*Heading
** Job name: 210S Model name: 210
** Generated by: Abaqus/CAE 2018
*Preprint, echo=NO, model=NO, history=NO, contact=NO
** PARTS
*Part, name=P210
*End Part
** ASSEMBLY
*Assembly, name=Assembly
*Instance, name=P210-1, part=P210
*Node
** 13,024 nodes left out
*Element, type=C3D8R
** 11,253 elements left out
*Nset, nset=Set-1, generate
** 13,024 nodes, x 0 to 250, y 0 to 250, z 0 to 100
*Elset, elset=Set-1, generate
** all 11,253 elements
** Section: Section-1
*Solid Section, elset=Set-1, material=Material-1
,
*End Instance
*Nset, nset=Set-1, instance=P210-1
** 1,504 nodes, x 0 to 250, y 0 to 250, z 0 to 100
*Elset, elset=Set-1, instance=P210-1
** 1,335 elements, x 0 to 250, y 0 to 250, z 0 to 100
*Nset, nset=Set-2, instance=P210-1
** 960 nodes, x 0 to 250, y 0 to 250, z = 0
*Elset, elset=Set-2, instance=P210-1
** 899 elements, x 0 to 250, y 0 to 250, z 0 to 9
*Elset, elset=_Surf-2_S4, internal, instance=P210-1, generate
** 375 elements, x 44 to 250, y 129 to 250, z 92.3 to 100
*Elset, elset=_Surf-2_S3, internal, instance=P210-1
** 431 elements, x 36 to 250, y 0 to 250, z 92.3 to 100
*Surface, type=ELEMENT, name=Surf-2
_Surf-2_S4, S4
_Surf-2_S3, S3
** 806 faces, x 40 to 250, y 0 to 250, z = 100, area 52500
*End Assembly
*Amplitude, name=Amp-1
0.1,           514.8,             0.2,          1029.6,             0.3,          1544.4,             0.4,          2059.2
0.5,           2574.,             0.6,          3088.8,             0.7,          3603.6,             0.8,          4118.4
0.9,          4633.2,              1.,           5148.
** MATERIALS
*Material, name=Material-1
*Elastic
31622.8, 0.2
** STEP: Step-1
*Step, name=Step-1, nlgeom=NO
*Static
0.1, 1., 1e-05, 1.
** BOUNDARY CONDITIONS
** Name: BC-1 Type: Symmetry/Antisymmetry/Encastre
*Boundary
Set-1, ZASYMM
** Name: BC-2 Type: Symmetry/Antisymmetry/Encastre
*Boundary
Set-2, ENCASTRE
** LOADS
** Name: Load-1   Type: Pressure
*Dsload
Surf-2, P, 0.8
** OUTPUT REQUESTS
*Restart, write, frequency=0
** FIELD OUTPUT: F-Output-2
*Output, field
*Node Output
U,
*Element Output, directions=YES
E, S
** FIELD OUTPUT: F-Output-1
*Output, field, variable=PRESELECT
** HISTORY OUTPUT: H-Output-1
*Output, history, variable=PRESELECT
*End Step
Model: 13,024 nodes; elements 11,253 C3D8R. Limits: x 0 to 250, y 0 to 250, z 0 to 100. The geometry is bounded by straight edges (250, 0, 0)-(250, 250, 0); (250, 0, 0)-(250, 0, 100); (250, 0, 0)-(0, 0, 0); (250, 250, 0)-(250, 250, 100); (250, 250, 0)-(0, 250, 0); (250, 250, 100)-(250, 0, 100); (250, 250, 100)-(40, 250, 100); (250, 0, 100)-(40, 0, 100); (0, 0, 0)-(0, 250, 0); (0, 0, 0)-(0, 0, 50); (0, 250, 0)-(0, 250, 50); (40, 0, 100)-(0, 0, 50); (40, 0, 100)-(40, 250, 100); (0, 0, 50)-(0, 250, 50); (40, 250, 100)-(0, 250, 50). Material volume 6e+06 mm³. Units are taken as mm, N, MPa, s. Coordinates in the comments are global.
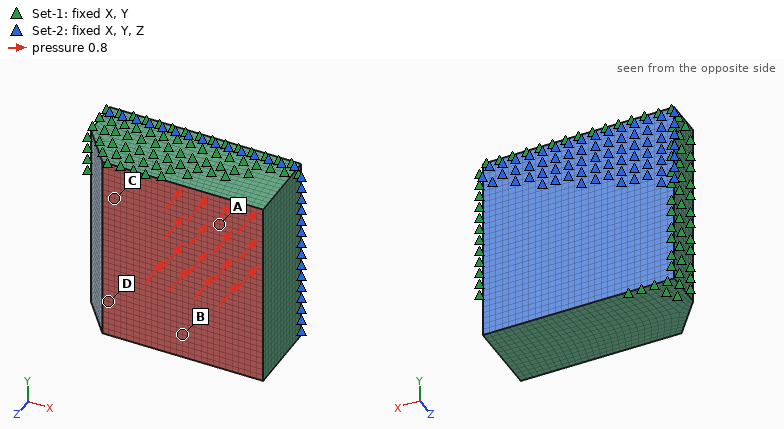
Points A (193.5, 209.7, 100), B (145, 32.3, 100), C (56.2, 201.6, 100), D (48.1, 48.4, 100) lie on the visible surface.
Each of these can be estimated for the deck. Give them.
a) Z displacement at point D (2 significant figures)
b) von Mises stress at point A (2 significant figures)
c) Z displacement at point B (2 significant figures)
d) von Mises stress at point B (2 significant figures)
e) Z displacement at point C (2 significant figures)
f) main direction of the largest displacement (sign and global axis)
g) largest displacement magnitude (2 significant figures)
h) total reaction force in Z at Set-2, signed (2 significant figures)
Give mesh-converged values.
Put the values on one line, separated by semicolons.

-0.0016 mm; 0.60 MPa; -0.0023 mm; 0.58 MPa; -0.0018 mm; -Z; 0.0023 mm; 42000 N
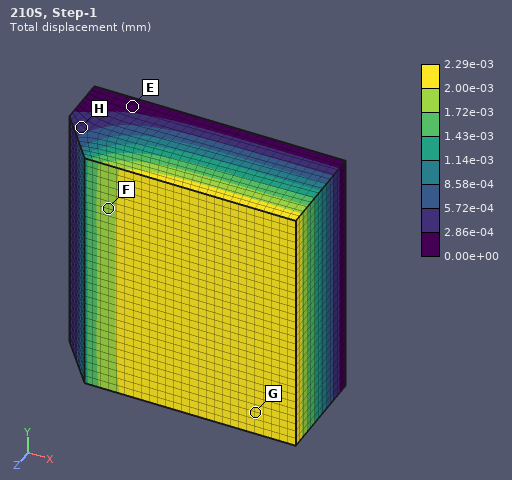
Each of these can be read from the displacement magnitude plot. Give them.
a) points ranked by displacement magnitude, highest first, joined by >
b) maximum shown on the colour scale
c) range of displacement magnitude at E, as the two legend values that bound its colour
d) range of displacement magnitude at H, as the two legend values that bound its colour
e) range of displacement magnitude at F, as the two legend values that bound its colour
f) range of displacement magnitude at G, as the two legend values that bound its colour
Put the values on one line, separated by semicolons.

G > F > H > E; 2.29e-03 mm; 0.00e+00 to 2.86e-04 mm; 2.86e-04 to 5.72e-04 mm; 1.72e-03 to 2.00e-03 mm; 2.00e-03 to 2.29e-03 mm
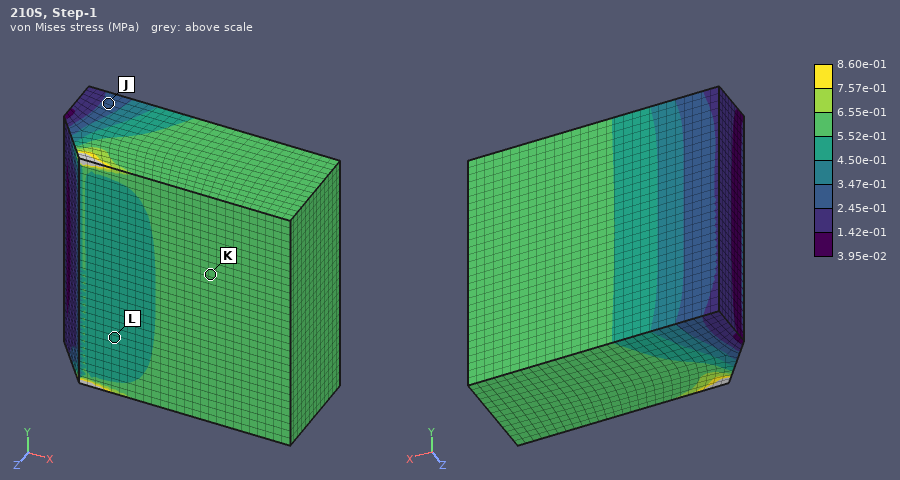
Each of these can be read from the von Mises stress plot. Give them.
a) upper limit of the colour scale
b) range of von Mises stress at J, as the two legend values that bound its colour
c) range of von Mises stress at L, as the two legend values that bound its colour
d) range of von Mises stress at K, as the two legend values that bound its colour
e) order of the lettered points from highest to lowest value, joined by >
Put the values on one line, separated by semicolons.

8.60e-01 MPa; 2.45e-01 to 3.47e-01 MPa; 4.50e-01 to 5.52e-01 MPa; 5.52e-01 to 6.55e-01 MPa; K > L > J
